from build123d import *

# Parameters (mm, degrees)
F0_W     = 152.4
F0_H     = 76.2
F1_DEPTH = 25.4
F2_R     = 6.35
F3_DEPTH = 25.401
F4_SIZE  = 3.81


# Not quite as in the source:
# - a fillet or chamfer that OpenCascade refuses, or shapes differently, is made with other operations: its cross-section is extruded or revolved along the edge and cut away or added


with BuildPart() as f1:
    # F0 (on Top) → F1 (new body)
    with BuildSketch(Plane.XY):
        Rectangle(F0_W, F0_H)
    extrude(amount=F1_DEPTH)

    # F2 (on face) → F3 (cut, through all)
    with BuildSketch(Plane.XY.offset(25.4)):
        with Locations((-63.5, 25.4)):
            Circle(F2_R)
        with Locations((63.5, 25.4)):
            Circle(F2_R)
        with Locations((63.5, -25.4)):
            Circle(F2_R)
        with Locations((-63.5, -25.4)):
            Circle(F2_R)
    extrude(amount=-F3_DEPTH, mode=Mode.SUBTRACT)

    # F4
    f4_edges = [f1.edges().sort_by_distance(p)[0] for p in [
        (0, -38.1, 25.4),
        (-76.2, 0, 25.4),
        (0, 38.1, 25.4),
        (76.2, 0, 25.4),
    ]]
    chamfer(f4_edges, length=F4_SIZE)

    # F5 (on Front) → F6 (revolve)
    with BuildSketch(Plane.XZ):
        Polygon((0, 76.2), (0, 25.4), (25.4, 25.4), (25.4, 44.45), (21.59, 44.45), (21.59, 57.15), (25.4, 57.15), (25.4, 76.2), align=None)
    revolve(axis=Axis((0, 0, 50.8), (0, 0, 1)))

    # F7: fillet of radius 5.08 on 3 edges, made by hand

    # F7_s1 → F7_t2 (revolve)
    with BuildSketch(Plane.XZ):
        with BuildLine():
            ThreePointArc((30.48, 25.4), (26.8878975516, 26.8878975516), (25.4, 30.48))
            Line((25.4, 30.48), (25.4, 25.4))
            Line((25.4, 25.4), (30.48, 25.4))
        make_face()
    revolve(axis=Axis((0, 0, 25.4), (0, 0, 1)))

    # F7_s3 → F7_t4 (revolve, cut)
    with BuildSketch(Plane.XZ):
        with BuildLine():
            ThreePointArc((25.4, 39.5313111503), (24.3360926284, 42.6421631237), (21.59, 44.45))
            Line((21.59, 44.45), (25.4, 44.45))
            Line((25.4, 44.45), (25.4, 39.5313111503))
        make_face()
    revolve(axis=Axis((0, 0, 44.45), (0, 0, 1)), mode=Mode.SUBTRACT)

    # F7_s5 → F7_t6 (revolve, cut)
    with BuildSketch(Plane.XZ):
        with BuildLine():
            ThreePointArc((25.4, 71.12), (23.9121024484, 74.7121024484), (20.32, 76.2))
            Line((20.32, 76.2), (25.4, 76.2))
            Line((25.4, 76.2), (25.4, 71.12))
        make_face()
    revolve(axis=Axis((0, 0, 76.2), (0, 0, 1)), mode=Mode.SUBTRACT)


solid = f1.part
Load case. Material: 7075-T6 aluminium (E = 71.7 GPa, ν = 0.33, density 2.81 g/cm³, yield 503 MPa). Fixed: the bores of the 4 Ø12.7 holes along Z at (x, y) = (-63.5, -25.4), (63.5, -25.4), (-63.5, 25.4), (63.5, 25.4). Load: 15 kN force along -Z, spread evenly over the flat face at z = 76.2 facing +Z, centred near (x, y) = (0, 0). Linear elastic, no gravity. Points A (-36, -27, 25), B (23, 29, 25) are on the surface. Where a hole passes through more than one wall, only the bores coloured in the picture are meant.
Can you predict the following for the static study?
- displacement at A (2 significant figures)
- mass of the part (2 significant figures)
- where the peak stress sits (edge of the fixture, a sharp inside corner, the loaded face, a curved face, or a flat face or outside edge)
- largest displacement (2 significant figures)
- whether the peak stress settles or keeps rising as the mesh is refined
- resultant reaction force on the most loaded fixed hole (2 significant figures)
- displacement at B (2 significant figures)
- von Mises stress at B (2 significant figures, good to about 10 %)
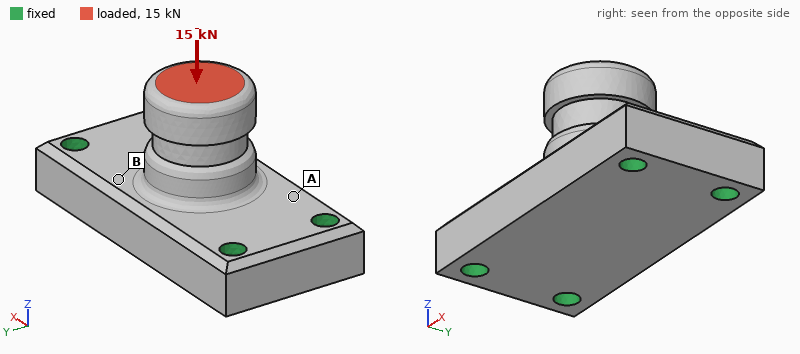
11 µm
1.1 kg
edge of the fixture
26 µm
keeps rising
3.9 kN
16 µm
9.1 MPa
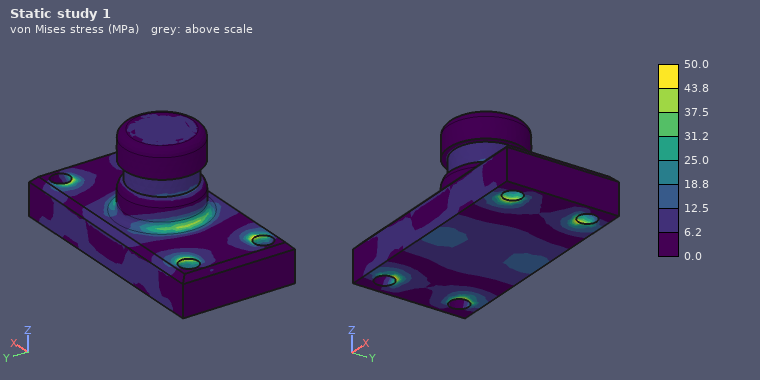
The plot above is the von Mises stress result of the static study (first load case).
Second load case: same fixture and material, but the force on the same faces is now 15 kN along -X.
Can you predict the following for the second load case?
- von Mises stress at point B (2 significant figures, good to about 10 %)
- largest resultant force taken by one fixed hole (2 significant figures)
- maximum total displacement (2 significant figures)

19 MPa
6.3 kN
0.10 mm
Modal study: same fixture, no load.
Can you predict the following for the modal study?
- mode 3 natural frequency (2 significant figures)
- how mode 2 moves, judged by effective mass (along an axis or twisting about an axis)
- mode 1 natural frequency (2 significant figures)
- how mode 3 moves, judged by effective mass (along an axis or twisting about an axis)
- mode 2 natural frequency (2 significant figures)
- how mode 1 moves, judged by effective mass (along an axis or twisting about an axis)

6300 Hz
along Z
4300 Hz
along X
5600 Hz
along Y
